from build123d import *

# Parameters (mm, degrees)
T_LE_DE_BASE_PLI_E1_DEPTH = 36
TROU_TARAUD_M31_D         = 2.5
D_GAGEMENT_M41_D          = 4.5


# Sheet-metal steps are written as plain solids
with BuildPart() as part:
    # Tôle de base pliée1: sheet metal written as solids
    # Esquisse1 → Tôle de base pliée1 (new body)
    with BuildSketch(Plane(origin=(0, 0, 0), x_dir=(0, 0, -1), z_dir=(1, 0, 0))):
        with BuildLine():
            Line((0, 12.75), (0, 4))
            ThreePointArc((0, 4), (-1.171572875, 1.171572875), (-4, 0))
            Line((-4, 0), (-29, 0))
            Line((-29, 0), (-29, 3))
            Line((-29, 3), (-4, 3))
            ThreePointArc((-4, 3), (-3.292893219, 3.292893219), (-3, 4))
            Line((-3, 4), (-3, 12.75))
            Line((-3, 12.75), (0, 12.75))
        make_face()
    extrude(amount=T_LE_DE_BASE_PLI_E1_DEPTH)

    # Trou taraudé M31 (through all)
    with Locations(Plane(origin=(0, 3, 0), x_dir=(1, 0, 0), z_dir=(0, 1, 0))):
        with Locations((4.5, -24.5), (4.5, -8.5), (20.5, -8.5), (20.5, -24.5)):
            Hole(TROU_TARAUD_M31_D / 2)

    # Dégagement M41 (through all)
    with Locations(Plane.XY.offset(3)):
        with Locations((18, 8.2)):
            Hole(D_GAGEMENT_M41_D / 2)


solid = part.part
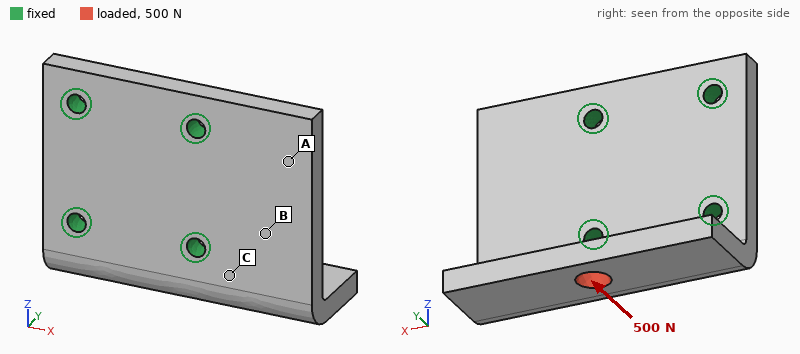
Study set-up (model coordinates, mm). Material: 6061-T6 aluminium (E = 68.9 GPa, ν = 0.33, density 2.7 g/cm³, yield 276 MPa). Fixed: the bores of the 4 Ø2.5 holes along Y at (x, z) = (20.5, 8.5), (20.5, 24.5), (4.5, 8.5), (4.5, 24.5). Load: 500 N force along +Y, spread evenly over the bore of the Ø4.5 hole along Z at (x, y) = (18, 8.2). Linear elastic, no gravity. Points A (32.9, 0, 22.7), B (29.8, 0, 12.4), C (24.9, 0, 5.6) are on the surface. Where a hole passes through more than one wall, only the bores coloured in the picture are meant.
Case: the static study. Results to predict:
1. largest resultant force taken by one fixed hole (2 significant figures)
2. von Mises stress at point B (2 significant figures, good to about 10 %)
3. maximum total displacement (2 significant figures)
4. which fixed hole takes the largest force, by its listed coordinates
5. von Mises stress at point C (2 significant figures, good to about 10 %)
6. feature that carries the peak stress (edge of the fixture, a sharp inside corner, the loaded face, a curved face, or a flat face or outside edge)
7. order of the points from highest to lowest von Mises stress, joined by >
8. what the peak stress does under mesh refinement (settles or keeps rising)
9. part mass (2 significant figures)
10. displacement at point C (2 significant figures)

450 N
19 MPa
43 µm
(20.5, 8.5)
37 MPa
edge of the fixture
C > B > A
keeps rising
11 g
9.1 µm
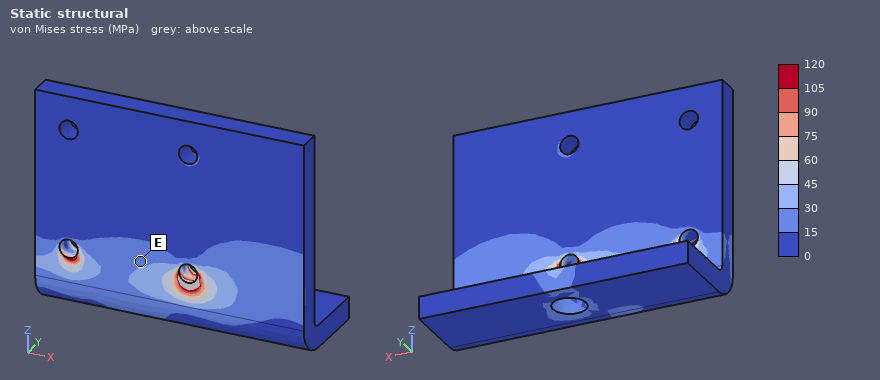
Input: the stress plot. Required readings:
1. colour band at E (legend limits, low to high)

15 to 30 MPa
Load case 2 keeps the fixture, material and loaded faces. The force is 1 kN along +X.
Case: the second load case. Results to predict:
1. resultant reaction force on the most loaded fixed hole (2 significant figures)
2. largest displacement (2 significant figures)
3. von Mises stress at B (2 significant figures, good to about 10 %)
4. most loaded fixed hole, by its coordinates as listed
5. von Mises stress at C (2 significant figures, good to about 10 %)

760 N
56 µm
24 MPa
(20.5, 8.5)
24 MPa
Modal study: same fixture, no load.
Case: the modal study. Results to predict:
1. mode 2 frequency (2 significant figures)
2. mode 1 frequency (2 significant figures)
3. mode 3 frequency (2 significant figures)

11 kHz
8800 Hz
12 kHz
